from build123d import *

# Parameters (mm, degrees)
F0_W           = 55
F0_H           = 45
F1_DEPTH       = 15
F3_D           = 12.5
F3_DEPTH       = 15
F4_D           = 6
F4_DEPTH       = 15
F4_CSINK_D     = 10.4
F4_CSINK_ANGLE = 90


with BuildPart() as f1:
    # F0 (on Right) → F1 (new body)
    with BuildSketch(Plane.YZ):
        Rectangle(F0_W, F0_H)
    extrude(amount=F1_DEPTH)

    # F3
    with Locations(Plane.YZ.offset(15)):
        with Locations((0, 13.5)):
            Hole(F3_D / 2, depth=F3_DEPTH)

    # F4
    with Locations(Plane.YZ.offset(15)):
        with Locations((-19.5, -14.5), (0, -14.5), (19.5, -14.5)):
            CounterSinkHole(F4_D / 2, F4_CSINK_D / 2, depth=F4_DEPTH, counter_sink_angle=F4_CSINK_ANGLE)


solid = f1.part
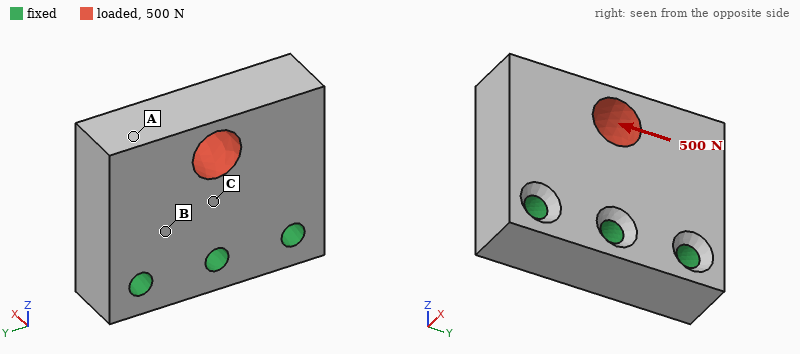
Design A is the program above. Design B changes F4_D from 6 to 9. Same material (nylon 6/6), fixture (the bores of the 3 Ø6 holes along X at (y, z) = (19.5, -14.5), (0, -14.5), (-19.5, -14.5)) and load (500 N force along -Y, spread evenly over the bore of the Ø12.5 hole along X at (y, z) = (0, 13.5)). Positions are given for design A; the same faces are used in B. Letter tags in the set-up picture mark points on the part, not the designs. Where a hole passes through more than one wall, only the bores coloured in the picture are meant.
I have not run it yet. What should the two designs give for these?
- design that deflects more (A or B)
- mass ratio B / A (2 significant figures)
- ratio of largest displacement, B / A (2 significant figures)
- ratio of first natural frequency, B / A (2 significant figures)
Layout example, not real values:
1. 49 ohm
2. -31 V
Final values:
1. A
2. 0.96
3. 0.88
4. 1.2
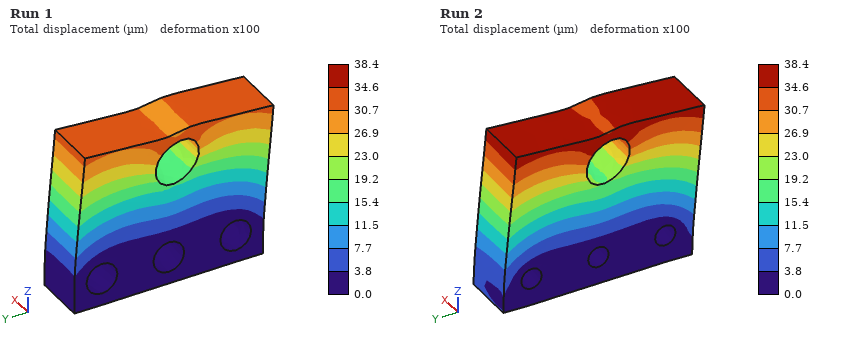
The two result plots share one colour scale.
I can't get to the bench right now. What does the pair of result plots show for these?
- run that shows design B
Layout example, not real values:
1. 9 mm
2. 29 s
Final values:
1. Run 1
